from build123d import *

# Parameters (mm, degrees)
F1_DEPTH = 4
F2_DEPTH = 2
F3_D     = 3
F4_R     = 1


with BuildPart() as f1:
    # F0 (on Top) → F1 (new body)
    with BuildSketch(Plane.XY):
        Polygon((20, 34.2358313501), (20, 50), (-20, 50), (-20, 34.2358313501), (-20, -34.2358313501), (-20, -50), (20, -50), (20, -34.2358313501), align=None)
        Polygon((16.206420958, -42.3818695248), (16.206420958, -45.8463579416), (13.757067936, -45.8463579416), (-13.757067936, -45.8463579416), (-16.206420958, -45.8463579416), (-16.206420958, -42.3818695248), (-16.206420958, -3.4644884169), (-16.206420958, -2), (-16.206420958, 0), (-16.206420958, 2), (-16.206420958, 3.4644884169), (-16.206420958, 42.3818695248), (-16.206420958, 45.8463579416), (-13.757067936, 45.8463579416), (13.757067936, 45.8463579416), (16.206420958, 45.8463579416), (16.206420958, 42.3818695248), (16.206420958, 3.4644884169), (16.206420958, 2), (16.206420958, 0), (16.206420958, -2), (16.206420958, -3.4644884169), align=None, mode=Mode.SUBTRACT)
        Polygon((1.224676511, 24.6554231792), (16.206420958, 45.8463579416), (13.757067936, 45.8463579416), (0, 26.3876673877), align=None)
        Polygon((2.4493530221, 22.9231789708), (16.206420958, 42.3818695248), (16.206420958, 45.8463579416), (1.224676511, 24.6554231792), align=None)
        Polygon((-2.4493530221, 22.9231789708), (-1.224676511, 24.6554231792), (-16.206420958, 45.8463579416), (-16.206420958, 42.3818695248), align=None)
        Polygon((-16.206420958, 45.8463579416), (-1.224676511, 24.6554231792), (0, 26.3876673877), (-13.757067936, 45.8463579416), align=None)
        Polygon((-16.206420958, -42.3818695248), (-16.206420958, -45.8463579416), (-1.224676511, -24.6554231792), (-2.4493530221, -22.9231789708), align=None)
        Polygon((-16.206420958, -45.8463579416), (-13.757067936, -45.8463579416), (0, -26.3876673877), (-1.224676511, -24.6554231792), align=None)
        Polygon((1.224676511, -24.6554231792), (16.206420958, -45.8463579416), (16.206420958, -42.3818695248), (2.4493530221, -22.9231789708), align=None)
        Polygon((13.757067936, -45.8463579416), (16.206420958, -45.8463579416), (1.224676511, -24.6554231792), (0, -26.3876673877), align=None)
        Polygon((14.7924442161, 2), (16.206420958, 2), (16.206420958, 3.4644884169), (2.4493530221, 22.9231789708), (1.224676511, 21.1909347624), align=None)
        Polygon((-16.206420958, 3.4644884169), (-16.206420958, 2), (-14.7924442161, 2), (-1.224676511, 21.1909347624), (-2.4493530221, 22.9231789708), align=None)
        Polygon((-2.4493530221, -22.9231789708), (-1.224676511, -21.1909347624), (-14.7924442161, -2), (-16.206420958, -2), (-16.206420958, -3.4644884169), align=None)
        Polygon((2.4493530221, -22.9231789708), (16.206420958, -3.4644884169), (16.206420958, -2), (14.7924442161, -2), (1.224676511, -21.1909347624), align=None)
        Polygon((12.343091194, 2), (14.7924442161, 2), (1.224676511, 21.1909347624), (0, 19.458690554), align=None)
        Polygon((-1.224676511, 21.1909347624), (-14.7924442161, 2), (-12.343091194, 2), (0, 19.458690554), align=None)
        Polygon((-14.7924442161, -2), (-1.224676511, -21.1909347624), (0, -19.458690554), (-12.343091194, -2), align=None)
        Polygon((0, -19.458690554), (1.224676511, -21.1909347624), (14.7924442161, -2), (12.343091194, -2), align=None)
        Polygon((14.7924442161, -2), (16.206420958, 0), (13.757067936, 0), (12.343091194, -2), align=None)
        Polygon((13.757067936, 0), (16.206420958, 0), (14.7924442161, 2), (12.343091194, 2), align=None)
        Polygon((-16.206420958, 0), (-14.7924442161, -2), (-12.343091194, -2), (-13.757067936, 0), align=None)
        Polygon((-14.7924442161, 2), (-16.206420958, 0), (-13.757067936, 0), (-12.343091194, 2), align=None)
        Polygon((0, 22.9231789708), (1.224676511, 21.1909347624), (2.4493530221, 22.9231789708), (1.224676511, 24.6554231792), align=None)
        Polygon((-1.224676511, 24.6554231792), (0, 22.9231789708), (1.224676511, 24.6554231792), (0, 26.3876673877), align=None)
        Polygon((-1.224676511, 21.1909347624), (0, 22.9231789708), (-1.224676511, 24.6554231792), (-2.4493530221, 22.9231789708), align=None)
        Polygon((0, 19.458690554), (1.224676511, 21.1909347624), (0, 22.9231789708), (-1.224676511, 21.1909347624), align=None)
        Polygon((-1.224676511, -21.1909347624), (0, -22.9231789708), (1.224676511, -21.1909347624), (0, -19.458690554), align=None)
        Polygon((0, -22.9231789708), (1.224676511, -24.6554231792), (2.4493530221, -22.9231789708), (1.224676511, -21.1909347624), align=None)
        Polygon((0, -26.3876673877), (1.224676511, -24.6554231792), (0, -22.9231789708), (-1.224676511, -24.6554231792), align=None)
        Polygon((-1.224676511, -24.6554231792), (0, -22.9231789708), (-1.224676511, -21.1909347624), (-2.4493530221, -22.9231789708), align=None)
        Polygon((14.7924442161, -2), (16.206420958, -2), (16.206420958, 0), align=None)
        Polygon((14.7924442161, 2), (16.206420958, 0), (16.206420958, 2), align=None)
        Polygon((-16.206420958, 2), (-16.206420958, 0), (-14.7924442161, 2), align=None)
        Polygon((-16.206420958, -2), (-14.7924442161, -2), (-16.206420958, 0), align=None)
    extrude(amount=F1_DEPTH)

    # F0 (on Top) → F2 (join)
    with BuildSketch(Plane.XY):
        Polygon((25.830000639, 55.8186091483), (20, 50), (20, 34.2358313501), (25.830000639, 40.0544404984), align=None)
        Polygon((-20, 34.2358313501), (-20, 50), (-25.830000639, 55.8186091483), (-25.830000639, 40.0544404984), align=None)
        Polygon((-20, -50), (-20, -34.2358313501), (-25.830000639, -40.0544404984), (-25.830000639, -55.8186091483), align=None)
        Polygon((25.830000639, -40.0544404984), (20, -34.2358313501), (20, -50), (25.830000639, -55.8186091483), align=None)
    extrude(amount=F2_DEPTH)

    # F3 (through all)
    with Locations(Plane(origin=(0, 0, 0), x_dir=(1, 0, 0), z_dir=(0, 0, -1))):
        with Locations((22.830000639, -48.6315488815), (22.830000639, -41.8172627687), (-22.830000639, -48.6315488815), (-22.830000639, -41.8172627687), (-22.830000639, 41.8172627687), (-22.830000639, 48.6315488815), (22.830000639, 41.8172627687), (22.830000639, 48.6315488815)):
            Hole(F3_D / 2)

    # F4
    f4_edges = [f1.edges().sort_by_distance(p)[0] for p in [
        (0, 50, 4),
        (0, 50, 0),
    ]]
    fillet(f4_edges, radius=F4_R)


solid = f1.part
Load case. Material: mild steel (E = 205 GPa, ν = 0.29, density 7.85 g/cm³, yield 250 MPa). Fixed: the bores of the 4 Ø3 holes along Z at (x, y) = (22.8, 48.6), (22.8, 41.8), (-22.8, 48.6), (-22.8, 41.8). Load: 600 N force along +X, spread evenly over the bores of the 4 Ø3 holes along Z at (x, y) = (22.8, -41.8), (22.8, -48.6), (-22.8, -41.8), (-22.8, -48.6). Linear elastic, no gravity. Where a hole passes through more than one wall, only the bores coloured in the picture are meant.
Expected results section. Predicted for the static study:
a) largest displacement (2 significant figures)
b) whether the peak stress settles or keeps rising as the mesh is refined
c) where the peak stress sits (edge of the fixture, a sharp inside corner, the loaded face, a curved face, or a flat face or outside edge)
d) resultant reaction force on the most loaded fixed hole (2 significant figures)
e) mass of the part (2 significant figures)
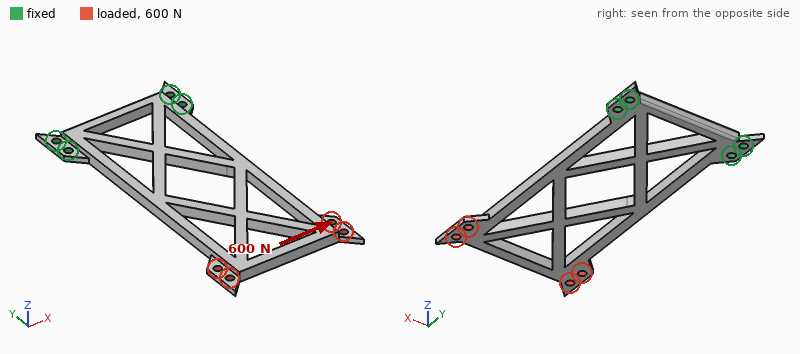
0.15 mm
keeps rising
edge of the fixture
960 N
63 g
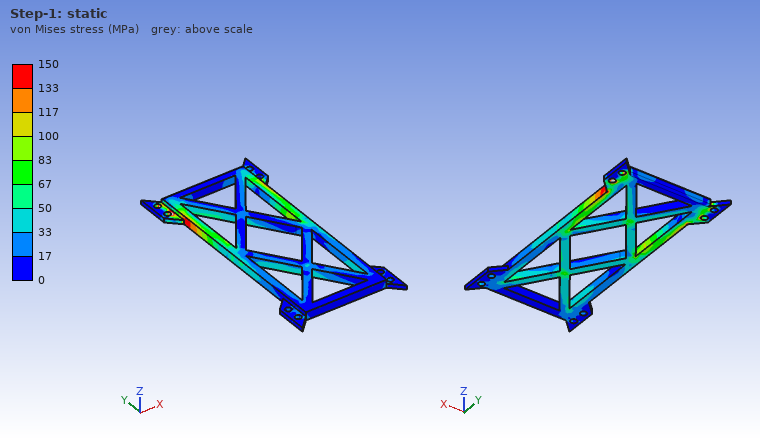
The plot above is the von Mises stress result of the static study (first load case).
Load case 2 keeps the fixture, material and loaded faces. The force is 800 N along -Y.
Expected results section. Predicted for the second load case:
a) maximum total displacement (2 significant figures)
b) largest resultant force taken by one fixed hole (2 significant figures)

0.25 mm
290 N
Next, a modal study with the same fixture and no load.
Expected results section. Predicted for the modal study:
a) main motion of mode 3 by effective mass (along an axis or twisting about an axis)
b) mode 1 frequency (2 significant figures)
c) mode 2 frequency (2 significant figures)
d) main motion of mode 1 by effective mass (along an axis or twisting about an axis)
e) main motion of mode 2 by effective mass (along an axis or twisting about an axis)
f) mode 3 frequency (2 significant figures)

along Z
280 Hz
1000 Hz
along Z
twisting about Y
1800 Hz
